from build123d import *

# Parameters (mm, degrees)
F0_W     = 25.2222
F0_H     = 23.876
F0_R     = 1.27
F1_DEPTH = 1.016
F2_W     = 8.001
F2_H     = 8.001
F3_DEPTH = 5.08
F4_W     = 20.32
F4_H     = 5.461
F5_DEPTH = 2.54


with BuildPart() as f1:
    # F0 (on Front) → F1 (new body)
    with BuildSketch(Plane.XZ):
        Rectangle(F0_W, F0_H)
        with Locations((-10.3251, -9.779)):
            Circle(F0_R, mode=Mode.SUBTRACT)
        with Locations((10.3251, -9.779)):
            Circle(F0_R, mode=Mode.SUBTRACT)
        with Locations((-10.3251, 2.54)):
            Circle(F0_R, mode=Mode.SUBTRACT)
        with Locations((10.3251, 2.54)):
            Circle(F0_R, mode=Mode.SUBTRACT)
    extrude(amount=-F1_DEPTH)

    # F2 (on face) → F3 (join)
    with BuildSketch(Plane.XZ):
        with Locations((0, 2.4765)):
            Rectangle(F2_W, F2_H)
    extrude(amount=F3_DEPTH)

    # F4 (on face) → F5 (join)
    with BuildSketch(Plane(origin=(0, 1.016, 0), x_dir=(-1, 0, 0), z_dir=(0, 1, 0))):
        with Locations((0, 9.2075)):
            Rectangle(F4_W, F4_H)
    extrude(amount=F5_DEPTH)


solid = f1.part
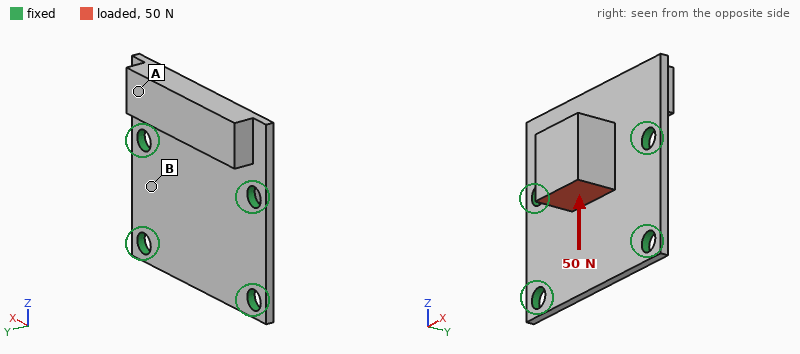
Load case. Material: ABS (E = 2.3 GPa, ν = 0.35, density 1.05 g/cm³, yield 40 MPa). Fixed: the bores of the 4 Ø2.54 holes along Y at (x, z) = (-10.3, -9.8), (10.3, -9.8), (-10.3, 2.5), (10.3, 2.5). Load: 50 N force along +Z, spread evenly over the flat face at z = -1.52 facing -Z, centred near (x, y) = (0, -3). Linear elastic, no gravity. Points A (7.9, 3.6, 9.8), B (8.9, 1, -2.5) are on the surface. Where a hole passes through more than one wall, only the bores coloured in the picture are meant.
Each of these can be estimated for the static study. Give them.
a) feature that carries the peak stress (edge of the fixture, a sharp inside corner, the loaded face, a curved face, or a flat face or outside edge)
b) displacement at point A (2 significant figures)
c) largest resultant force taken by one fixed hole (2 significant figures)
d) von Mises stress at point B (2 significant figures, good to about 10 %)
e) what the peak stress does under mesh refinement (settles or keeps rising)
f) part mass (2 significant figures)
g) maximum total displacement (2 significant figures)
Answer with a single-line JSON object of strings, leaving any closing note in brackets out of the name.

{"feature that carries the peak stress": "edge of the fixture", "displacement at point A": "0.19 mm", "largest resultant force taken by one fixed hole": "18 N", "von Mises stress at point B": "5.1 MPa", "what the peak stress does under mesh refinement": "keeps rising", "part mass": "1.3 g", "maximum total displacement": "0.26 mm"}
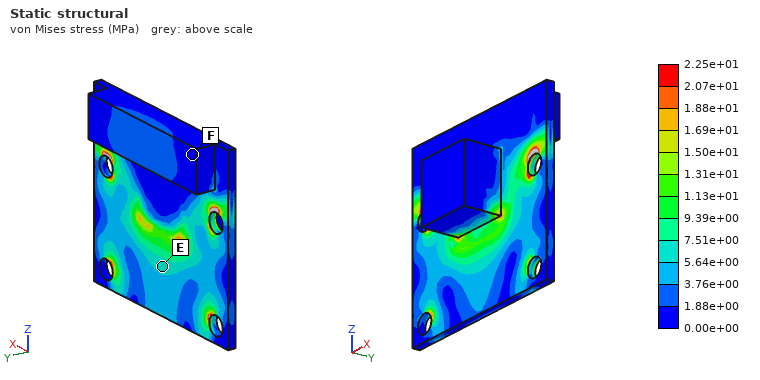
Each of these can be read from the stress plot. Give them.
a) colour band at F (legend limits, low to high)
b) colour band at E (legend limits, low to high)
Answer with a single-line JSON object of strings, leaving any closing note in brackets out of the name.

{"colour band at F": "0.00e+00 to 1.88e+00 MPa", "colour band at E": "5.64e+00 to 7.51e+00 MPa"}
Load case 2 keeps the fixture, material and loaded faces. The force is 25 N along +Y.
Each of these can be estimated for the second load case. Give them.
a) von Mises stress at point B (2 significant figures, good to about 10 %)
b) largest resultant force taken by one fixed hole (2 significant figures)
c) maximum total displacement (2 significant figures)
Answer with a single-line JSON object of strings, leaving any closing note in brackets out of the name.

{"von Mises stress at point B": "5.9 MPa", "largest resultant force taken by one fixed hole": "9.1 N", "maximum total displacement": "0.21 mm"}
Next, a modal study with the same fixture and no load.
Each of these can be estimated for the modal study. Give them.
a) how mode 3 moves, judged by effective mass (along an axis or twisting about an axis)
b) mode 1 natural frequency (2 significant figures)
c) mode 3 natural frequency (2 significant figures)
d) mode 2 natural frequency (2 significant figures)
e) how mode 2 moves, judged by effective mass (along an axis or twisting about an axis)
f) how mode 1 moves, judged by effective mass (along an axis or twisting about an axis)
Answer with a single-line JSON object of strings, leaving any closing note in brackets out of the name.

{"how mode 3 moves, judged by effective mass": "twisting about Z", "mode 1 natural frequency": "1900 Hz", "mode 3 natural frequency": "5500 Hz", "mode 2 natural frequency": "3600 Hz", "how mode 2 moves, judged by effective mass": "along Y", "how mode 1 moves, judged by effective mass": "along Y"}
